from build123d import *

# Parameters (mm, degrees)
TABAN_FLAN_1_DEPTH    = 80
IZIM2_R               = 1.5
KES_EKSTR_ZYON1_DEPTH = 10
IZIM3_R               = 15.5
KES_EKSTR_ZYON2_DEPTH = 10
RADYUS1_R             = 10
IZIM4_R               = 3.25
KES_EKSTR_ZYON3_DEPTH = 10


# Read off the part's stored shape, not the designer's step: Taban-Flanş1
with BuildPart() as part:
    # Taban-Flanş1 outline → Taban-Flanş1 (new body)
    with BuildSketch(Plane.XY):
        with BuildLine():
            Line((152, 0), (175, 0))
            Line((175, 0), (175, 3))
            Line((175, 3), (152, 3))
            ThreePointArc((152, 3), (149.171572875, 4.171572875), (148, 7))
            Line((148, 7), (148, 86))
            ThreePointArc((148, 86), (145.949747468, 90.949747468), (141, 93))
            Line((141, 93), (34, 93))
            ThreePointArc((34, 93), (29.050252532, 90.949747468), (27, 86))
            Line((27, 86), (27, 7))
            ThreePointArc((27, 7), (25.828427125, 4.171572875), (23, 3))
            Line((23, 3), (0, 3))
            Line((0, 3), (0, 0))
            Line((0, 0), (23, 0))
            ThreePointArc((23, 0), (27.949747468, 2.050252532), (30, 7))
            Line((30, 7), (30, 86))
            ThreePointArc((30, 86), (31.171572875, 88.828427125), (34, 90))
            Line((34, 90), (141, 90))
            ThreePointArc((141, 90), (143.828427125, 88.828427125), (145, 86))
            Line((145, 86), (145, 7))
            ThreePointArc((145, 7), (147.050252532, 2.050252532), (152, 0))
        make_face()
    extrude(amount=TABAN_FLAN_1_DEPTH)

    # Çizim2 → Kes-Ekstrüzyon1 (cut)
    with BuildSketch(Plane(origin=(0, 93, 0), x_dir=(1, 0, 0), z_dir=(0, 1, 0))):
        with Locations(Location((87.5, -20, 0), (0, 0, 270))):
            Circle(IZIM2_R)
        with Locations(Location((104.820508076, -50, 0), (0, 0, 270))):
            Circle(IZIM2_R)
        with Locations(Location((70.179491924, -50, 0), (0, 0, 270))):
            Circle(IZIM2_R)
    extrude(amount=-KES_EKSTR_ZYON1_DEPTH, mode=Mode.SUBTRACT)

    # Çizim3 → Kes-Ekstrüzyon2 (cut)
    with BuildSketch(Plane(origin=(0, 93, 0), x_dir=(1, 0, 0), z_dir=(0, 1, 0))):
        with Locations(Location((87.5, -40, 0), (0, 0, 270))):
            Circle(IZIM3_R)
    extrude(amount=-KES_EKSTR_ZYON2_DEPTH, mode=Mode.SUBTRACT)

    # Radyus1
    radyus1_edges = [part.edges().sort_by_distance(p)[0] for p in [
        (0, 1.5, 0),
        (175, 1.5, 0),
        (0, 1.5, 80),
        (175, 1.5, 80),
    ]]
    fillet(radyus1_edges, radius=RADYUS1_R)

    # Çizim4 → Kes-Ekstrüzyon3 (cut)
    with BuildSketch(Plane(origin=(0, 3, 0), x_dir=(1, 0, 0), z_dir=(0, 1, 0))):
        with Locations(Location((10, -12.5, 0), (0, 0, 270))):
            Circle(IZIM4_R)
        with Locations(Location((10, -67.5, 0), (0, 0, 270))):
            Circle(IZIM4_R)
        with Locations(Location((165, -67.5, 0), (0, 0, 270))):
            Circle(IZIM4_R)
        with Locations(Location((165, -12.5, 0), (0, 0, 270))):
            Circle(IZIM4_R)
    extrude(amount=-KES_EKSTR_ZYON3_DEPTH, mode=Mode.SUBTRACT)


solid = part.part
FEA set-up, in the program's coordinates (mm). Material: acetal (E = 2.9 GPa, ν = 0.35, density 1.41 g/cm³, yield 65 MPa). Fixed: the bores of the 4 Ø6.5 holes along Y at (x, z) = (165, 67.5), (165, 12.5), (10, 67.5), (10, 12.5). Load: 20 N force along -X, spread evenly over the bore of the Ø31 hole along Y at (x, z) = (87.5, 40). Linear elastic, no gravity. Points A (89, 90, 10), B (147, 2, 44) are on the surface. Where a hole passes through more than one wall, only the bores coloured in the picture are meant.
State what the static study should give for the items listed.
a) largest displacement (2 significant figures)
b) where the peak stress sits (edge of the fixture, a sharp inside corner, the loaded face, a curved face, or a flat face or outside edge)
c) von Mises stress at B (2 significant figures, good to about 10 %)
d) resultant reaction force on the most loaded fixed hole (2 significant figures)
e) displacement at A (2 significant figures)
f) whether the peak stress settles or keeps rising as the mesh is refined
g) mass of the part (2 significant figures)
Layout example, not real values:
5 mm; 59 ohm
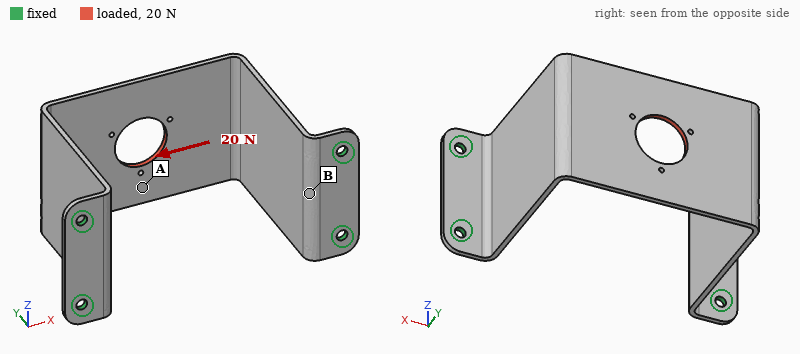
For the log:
2.1 mm; edge of the fixture; 2.7 MPa; 6.7 N; 2.1 mm; keeps rising; 110 g
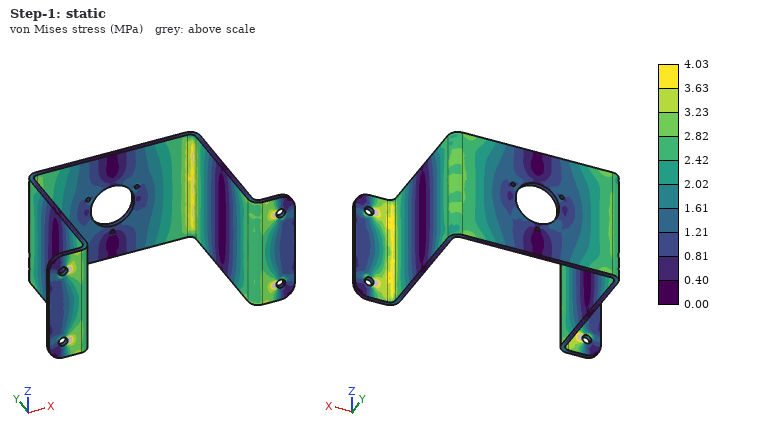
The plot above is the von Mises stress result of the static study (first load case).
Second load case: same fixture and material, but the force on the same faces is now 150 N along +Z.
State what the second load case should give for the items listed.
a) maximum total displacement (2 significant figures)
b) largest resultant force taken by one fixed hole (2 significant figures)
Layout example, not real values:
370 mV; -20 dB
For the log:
2.1 mm; 130 N
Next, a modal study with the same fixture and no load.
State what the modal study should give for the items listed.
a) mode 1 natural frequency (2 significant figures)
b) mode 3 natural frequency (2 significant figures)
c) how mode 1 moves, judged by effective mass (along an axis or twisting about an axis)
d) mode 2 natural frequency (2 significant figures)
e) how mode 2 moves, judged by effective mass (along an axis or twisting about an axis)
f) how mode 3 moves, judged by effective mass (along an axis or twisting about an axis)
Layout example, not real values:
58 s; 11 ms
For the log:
65 Hz; 200 Hz; along X; 180 Hz; along Z; twisting about Y
